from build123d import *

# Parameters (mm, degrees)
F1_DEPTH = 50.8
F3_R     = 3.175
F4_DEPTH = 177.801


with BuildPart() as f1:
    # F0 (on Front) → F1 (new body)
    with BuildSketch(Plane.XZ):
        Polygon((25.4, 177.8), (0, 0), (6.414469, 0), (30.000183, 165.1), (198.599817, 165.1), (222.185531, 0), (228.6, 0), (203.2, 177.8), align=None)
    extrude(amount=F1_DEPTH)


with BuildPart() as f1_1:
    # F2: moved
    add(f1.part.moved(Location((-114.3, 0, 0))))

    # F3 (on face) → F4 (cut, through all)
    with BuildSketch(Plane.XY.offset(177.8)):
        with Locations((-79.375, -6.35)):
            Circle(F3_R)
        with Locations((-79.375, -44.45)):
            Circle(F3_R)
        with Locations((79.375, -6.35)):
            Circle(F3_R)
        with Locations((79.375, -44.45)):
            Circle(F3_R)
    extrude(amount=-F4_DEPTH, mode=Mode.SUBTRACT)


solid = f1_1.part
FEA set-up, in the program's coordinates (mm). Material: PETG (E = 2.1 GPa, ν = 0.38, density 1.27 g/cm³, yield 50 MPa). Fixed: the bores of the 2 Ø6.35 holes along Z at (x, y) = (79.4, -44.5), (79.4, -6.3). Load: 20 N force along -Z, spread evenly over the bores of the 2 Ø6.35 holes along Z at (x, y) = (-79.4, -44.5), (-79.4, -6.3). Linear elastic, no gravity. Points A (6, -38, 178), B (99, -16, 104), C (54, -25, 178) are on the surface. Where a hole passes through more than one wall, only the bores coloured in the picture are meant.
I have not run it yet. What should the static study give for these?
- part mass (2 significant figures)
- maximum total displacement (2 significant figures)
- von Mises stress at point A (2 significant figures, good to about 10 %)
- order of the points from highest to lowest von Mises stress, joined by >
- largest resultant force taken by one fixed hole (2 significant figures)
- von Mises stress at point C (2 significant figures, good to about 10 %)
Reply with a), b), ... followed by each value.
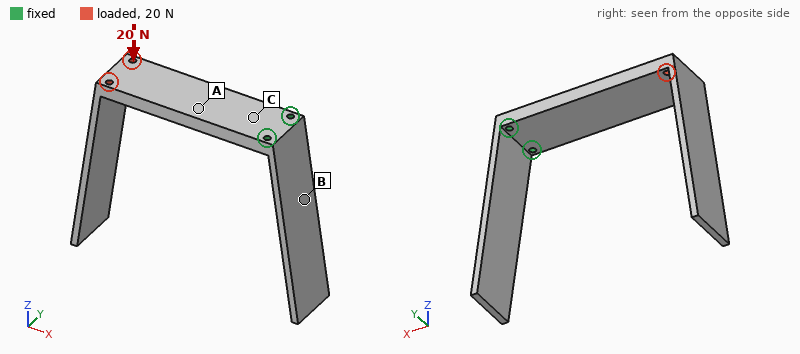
a) 280 g
b) 3.1 mm
c) 1.3 MPa
d) C > A > B
e) 10 N
f) 1.8 MPa
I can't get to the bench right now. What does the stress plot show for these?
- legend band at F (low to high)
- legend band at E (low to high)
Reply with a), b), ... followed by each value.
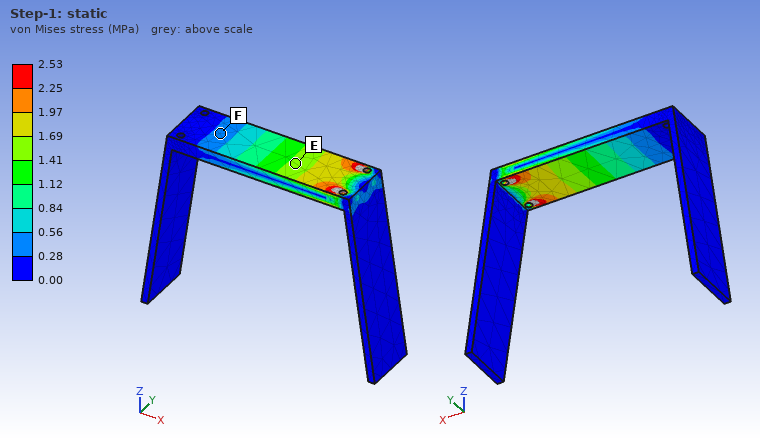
a) 0.28 to 0.56 MPa
b) 1.41 to 1.69 MPa
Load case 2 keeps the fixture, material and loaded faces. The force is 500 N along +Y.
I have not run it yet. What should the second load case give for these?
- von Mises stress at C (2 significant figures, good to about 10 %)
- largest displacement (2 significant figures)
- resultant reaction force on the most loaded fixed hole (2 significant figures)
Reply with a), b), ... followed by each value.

a) 2.0 MPa
b) 3.2 mm
c) 2.0 kN
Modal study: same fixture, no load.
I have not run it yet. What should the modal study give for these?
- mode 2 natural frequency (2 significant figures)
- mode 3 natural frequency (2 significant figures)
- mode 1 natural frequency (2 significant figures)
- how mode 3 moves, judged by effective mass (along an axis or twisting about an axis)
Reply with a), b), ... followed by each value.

a) 46 Hz
b) 67 Hz
c) 33 Hz
d) along Y
